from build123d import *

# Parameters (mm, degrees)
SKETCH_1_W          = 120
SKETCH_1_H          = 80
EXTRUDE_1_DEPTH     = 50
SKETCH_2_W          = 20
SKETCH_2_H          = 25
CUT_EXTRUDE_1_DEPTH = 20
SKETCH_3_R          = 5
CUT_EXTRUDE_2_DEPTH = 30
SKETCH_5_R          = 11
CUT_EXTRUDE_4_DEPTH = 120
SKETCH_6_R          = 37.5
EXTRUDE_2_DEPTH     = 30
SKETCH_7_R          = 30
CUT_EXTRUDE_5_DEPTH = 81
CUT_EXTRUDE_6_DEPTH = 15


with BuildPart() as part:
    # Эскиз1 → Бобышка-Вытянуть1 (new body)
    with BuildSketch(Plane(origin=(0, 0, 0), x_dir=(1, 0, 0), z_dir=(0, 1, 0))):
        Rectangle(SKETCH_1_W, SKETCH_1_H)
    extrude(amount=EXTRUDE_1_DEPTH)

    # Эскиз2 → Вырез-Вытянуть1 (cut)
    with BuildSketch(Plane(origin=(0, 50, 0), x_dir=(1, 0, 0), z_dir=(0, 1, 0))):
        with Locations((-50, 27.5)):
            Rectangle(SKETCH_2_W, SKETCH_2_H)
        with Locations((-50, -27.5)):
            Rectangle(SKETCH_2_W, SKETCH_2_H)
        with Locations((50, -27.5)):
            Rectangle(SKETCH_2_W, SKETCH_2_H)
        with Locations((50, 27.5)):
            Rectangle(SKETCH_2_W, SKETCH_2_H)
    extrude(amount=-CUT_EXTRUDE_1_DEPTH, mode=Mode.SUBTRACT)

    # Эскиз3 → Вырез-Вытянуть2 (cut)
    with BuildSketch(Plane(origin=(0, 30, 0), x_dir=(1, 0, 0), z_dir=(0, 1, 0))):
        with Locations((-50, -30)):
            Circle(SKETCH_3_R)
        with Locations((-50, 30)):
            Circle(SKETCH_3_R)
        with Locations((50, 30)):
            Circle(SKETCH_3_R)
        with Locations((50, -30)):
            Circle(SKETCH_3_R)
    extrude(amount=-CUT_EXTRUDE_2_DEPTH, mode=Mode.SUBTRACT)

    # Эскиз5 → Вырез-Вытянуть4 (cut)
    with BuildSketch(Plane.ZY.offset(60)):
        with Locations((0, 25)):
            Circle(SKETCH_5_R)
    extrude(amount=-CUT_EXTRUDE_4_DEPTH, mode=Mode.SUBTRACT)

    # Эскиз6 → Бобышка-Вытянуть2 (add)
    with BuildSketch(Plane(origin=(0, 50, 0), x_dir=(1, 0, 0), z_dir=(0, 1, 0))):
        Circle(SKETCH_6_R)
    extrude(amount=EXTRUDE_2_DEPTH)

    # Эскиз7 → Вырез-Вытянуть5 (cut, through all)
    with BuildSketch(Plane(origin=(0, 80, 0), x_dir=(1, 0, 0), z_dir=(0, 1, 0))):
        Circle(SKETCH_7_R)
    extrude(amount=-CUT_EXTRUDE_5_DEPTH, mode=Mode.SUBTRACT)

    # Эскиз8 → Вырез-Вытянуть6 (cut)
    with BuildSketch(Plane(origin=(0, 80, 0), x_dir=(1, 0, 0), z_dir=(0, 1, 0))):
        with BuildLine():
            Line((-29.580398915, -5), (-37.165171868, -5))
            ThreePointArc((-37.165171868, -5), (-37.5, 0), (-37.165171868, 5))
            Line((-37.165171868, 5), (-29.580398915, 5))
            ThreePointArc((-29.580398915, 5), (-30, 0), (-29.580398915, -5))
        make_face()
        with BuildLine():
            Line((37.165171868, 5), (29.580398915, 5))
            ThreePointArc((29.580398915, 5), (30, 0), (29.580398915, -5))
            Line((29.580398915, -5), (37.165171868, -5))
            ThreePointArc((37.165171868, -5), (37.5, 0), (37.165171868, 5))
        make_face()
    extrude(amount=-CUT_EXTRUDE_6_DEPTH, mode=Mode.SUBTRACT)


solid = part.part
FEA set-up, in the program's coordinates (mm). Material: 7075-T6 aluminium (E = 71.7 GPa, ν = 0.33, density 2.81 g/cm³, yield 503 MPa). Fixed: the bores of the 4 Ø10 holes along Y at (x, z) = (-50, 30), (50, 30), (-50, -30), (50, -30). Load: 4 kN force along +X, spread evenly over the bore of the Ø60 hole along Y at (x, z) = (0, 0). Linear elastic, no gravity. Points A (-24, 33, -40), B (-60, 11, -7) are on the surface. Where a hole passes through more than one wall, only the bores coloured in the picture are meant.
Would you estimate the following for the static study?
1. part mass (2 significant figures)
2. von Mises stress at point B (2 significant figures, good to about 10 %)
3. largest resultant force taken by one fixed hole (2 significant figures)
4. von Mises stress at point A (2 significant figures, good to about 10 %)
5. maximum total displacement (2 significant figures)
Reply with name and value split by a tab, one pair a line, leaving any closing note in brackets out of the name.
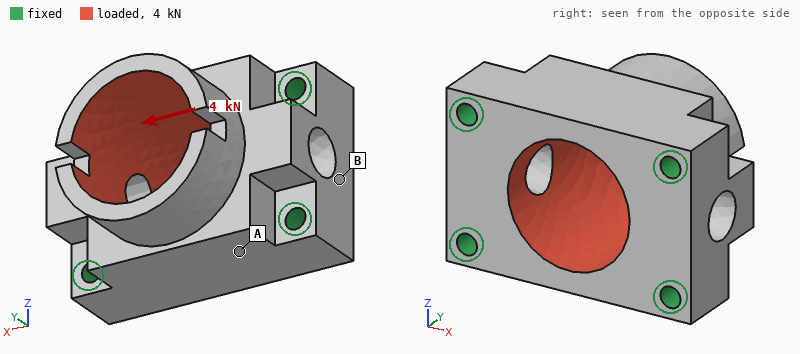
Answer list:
part mass	880 g
von Mises stress at point B	0.59 MPa
largest resultant force taken by one fixed hole	1.1 kN
von Mises stress at point A	1.4 MPa
maximum total displacement	5.5 µm
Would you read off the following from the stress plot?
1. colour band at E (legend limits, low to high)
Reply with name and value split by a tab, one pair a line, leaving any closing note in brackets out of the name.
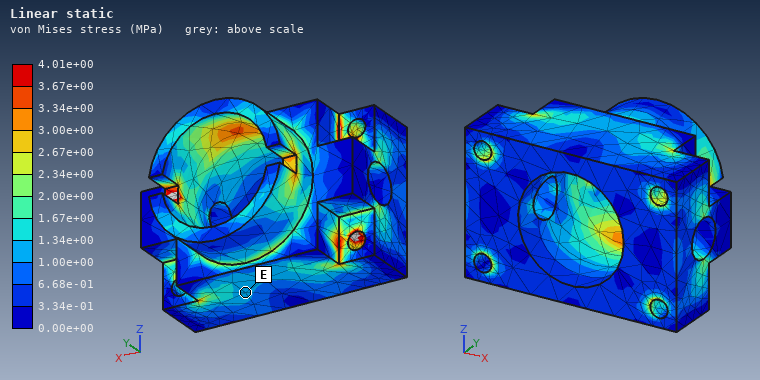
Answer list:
colour band at E	1.00e+00 to 1.34e+00 MPa
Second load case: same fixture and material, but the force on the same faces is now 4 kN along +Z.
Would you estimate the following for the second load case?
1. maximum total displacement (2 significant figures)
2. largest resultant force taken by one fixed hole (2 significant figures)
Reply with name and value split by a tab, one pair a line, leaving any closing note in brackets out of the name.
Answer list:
maximum total displacement	6.7 µm
largest resultant force taken by one fixed hole	1.3 kN
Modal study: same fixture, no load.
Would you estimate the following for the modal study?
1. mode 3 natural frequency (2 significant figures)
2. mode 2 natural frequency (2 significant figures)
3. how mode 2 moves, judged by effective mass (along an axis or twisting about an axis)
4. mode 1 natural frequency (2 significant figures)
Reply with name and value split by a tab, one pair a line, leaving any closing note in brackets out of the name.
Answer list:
mode 3 natural frequency	8800 Hz
mode 2 natural frequency	7600 Hz
how mode 2 moves, judged by effective mass	along Z
mode 1 natural frequency	7200 Hz
